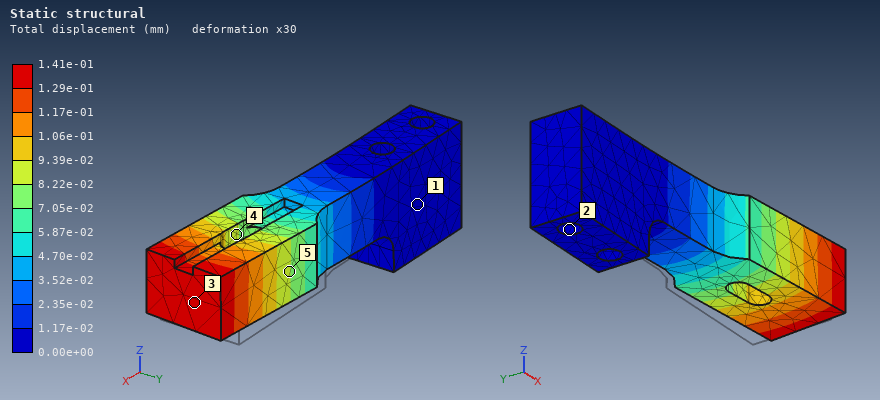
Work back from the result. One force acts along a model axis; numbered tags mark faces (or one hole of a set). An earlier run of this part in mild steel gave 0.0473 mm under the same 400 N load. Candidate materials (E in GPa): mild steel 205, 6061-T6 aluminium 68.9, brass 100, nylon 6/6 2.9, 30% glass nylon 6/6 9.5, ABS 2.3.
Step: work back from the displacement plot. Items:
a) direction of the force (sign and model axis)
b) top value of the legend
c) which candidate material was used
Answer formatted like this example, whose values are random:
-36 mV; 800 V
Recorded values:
-Y; 1.41e-01 mm; 6061-T6 aluminium
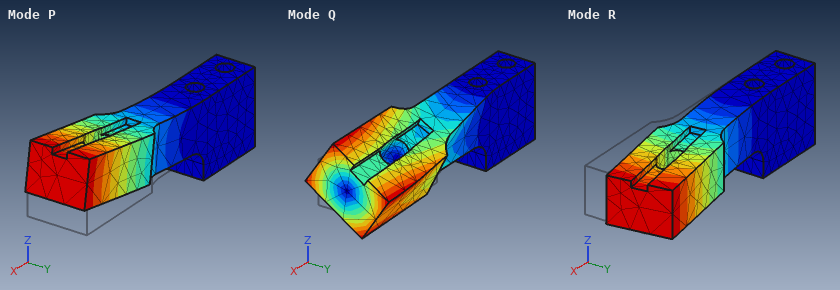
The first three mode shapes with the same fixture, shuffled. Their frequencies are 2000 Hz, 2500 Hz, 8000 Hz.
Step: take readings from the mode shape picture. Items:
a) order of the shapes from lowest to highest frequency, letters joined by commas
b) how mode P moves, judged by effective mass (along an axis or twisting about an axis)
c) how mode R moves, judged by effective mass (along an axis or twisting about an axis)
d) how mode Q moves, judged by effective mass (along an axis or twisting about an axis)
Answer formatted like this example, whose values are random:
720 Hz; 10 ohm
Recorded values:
R, P, Q; along Z; along Y; twisting about X
